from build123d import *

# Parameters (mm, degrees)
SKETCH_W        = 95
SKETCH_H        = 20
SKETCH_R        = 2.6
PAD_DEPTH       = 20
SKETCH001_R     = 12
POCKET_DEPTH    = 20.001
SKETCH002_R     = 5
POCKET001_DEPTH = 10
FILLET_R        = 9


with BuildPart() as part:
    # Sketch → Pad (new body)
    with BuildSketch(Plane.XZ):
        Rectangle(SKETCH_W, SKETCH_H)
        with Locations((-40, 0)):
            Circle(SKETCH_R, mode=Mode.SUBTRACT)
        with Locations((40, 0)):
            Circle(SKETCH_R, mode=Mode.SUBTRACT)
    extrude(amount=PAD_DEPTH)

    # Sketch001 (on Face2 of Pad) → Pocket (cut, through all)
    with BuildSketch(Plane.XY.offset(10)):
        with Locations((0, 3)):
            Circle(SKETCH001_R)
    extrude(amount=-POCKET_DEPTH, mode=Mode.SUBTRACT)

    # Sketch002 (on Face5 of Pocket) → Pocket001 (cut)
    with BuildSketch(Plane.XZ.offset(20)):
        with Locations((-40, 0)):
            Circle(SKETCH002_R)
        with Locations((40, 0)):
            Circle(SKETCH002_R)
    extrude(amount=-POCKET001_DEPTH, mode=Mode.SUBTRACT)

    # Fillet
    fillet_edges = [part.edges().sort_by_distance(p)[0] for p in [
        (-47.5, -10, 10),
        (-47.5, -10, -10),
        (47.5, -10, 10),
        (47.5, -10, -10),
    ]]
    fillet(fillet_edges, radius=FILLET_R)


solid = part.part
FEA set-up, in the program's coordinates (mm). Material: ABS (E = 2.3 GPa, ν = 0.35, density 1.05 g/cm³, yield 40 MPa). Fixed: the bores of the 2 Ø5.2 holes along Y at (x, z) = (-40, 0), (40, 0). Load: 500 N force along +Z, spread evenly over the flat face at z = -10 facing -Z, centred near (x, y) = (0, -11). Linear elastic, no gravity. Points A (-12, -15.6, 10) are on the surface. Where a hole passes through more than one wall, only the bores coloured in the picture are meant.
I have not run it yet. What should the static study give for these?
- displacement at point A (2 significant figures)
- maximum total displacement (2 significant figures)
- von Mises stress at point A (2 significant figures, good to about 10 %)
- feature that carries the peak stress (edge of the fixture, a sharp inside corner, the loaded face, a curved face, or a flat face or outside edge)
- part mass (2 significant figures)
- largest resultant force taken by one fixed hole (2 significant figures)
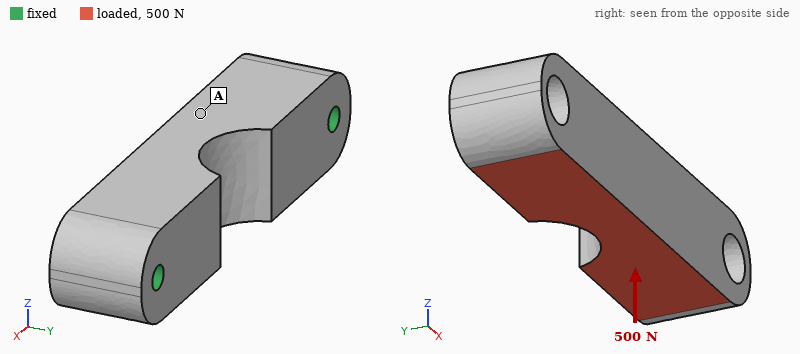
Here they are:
0.11 mm
0.13 mm
2.7 MPa
edge of the fixture
33 g
250 N
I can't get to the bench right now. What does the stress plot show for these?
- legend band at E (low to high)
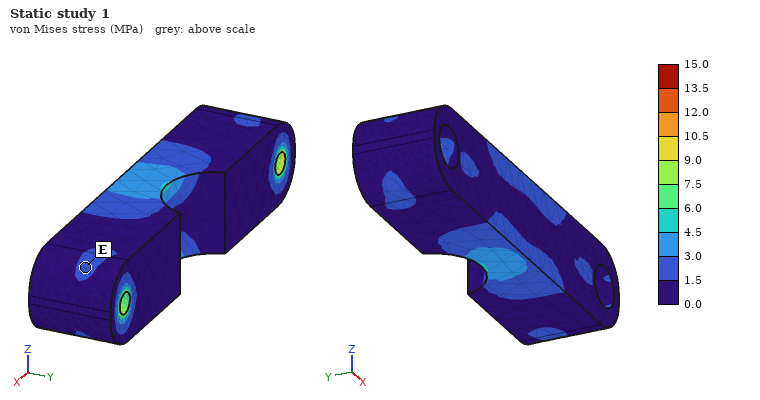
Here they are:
1.5 to 3.0 MPa
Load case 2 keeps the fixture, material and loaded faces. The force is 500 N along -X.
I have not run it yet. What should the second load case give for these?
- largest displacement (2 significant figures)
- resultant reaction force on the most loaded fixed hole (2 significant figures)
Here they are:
18 µm
260 N
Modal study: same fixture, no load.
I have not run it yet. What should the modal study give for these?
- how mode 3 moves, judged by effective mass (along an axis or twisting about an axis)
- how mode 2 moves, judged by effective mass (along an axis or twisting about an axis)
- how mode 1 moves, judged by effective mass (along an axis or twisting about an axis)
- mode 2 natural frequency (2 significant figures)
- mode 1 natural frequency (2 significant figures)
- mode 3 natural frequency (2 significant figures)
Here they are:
twisting about X
along Y
along Z
2700 Hz
2200 Hz
4200 Hz
